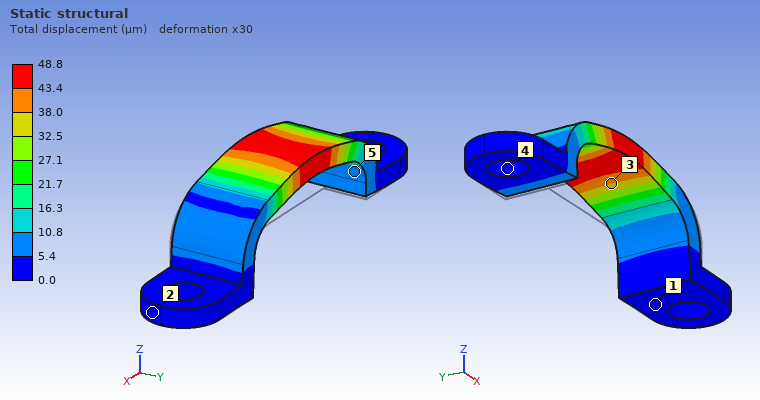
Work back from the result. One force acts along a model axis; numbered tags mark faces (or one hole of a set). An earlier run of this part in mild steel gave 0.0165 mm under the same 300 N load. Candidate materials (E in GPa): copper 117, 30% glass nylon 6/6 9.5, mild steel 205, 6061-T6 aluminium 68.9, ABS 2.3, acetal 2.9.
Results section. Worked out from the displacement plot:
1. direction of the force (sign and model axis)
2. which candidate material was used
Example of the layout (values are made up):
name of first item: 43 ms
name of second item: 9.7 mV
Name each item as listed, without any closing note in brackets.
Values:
direction of the force: +Z
which candidate material was used: 6061-T6 aluminium
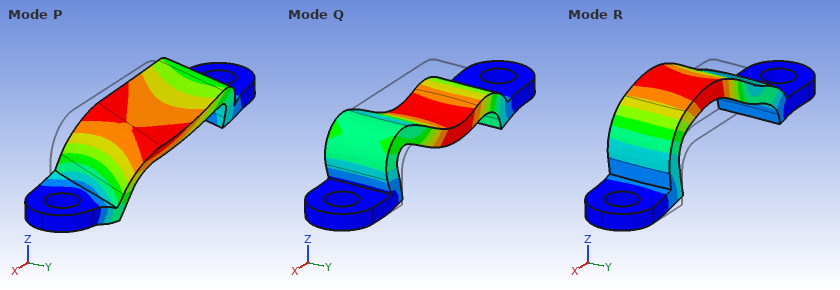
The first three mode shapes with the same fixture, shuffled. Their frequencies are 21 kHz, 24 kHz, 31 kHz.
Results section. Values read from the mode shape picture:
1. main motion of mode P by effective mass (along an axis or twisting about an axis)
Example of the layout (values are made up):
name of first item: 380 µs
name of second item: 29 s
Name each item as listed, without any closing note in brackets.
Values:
main motion of mode P by effective mass: along Y
